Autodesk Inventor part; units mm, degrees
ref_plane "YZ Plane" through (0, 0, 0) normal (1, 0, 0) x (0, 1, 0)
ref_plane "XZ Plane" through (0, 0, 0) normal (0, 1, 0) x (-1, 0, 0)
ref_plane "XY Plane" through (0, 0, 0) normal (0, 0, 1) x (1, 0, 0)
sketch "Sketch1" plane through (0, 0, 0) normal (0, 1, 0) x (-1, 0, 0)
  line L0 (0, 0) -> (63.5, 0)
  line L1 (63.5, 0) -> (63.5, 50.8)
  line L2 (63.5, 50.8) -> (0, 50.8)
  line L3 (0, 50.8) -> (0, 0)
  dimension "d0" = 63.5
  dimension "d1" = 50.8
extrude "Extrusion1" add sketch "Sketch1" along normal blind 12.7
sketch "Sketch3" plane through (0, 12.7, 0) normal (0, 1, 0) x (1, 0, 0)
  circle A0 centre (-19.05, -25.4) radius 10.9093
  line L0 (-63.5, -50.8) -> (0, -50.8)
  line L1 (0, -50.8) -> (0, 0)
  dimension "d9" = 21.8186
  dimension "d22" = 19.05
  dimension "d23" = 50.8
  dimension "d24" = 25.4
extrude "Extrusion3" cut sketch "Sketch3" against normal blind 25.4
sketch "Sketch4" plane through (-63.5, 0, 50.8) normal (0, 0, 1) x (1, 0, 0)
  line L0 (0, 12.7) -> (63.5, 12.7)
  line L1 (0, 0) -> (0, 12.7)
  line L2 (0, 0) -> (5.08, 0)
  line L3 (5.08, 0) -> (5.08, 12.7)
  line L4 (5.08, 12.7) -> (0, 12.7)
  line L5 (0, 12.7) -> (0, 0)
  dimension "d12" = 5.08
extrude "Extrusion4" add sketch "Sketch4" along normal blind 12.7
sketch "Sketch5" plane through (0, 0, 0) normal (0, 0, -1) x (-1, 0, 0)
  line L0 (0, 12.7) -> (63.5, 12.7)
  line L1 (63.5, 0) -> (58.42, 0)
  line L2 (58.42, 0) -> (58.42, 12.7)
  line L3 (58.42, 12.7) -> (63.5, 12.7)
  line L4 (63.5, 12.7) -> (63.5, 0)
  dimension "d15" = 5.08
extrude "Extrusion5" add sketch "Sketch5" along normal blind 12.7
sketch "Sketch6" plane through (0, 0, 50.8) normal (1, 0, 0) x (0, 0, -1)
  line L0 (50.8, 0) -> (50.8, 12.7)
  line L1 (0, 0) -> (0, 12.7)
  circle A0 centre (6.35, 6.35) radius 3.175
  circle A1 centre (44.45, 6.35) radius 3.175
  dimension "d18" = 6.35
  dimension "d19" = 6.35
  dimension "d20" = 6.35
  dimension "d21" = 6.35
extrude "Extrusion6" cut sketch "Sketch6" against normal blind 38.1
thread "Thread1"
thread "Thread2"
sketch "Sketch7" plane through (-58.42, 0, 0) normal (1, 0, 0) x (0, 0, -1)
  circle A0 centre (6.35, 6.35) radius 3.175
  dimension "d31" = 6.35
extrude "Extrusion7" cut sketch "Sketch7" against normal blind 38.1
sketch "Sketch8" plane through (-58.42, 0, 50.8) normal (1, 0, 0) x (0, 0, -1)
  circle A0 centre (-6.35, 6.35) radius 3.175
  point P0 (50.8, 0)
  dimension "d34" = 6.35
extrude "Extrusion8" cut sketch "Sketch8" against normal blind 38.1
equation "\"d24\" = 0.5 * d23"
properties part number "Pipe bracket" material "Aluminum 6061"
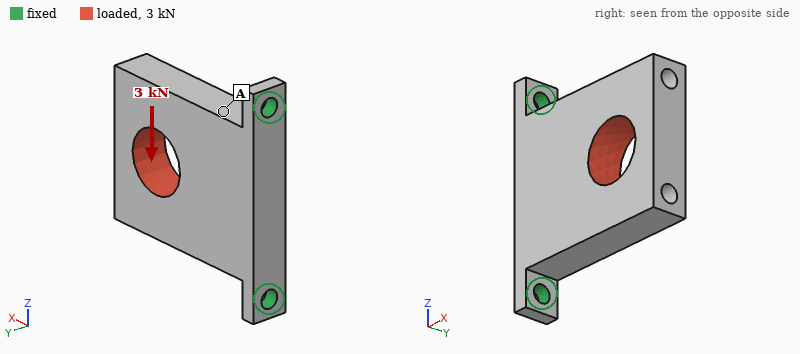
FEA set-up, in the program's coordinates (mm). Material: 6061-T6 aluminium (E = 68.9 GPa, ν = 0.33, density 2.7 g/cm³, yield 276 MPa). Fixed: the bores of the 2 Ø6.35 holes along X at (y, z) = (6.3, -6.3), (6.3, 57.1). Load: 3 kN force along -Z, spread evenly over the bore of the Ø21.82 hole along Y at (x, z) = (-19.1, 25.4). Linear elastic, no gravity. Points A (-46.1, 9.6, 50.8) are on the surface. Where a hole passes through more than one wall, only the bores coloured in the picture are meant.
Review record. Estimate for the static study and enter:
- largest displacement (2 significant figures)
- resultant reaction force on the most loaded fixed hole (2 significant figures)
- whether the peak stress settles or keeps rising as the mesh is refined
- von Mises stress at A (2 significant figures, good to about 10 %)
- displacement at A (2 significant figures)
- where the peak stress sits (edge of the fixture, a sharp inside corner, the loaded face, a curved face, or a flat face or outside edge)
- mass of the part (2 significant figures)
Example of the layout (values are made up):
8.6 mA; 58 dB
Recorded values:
73 µm; 2.8 kN; keeps rising; 20 MPa; 23 µm; edge of the fixture; 95 g
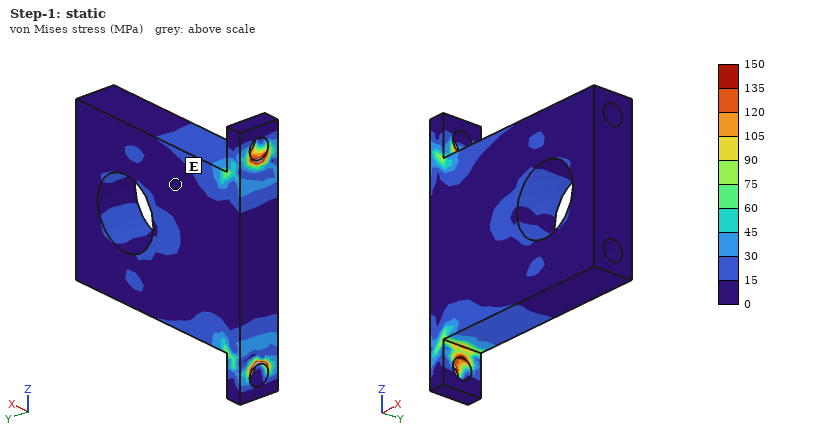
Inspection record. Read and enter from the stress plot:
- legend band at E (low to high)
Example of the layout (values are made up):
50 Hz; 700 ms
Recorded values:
0 to 15 MPa
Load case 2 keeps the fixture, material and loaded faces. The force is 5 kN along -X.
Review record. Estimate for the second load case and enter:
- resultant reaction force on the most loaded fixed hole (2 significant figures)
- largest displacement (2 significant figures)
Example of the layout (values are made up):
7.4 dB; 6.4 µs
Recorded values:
2.8 kN; 33 µm
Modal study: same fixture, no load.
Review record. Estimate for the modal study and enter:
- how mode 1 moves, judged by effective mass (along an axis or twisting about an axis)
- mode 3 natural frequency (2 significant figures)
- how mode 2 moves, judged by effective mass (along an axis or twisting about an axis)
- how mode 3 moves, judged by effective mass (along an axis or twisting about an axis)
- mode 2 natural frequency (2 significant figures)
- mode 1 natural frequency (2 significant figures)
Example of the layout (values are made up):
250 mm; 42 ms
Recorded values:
along Y; 5600 Hz; along Z; twisting about X; 5200 Hz; 1000 Hz
